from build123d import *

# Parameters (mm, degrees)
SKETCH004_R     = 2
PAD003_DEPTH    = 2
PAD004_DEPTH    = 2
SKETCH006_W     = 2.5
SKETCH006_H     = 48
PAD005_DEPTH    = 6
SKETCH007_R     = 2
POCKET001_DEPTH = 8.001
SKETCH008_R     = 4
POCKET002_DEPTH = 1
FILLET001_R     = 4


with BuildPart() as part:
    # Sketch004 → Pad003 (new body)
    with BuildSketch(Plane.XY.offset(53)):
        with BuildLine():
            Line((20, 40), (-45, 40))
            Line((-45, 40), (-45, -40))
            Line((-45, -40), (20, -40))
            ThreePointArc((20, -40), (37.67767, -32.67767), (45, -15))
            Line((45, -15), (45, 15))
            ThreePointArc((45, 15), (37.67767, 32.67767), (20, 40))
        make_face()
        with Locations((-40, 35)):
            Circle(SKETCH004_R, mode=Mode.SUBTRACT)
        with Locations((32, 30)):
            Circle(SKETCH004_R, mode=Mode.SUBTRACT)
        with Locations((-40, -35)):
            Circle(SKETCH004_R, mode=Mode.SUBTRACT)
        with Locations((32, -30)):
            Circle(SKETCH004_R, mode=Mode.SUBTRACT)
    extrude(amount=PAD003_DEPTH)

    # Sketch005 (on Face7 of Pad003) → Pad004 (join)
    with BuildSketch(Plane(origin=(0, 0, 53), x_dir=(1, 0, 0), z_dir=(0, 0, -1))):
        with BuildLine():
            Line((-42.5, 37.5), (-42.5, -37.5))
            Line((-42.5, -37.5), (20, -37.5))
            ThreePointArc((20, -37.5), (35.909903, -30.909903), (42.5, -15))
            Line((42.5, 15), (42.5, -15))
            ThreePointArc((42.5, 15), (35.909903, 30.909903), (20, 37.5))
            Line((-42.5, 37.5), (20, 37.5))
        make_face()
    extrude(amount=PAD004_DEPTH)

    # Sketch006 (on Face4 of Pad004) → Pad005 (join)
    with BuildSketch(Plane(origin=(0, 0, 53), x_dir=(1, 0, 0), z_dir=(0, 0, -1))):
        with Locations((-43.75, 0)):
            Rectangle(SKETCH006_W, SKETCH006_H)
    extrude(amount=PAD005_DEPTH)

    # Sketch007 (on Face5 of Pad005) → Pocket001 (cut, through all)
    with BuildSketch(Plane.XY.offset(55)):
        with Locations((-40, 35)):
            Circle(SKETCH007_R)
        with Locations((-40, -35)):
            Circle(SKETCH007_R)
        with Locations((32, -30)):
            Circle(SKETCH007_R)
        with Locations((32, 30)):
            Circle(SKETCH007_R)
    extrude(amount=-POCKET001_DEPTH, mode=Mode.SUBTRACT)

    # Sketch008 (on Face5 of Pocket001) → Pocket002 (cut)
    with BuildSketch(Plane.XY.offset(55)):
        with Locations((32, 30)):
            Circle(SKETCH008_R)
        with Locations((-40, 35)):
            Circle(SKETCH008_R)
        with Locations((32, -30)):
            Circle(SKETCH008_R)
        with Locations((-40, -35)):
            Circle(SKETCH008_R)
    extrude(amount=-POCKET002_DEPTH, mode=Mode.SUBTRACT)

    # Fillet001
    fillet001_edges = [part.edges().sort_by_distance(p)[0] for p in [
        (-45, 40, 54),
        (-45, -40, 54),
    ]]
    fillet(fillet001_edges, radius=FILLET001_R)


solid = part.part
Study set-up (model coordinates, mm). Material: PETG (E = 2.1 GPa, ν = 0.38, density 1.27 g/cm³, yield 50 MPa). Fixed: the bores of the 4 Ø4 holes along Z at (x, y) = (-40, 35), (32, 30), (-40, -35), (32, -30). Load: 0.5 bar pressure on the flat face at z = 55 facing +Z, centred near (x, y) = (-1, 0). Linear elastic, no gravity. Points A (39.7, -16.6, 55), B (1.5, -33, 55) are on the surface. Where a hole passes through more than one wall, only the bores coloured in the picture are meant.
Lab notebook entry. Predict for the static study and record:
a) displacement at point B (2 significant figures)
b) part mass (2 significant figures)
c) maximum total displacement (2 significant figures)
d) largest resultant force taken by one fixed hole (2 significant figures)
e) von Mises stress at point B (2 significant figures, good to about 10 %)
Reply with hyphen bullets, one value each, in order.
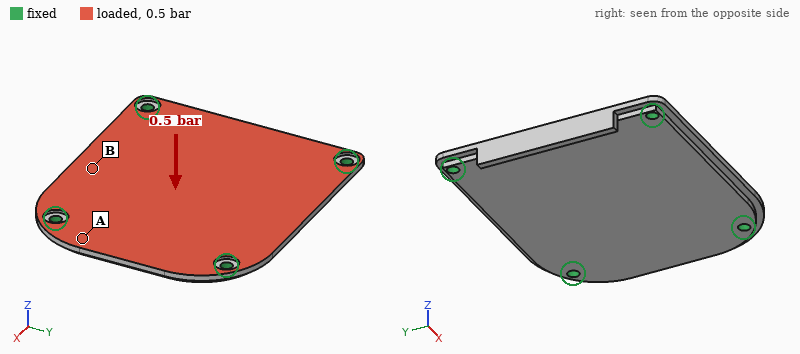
- 0.57 mm
- 34 g
- 0.81 mm
- 110 N
- 6.1 MPa
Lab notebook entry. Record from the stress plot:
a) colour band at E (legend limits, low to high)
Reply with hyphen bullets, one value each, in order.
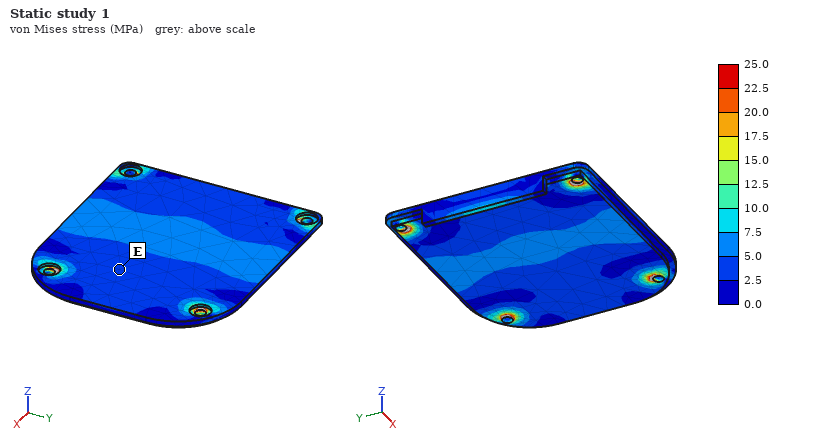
- 2.5 to 5.0 MPa
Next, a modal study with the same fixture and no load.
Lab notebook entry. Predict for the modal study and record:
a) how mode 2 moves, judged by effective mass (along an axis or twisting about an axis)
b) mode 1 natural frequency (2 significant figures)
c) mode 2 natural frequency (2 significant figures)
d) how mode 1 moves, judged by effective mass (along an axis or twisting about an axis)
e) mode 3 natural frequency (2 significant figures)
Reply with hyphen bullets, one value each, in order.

- twisting about X
- 660 Hz
- 1000 Hz
- along Z
- 1200 Hz
